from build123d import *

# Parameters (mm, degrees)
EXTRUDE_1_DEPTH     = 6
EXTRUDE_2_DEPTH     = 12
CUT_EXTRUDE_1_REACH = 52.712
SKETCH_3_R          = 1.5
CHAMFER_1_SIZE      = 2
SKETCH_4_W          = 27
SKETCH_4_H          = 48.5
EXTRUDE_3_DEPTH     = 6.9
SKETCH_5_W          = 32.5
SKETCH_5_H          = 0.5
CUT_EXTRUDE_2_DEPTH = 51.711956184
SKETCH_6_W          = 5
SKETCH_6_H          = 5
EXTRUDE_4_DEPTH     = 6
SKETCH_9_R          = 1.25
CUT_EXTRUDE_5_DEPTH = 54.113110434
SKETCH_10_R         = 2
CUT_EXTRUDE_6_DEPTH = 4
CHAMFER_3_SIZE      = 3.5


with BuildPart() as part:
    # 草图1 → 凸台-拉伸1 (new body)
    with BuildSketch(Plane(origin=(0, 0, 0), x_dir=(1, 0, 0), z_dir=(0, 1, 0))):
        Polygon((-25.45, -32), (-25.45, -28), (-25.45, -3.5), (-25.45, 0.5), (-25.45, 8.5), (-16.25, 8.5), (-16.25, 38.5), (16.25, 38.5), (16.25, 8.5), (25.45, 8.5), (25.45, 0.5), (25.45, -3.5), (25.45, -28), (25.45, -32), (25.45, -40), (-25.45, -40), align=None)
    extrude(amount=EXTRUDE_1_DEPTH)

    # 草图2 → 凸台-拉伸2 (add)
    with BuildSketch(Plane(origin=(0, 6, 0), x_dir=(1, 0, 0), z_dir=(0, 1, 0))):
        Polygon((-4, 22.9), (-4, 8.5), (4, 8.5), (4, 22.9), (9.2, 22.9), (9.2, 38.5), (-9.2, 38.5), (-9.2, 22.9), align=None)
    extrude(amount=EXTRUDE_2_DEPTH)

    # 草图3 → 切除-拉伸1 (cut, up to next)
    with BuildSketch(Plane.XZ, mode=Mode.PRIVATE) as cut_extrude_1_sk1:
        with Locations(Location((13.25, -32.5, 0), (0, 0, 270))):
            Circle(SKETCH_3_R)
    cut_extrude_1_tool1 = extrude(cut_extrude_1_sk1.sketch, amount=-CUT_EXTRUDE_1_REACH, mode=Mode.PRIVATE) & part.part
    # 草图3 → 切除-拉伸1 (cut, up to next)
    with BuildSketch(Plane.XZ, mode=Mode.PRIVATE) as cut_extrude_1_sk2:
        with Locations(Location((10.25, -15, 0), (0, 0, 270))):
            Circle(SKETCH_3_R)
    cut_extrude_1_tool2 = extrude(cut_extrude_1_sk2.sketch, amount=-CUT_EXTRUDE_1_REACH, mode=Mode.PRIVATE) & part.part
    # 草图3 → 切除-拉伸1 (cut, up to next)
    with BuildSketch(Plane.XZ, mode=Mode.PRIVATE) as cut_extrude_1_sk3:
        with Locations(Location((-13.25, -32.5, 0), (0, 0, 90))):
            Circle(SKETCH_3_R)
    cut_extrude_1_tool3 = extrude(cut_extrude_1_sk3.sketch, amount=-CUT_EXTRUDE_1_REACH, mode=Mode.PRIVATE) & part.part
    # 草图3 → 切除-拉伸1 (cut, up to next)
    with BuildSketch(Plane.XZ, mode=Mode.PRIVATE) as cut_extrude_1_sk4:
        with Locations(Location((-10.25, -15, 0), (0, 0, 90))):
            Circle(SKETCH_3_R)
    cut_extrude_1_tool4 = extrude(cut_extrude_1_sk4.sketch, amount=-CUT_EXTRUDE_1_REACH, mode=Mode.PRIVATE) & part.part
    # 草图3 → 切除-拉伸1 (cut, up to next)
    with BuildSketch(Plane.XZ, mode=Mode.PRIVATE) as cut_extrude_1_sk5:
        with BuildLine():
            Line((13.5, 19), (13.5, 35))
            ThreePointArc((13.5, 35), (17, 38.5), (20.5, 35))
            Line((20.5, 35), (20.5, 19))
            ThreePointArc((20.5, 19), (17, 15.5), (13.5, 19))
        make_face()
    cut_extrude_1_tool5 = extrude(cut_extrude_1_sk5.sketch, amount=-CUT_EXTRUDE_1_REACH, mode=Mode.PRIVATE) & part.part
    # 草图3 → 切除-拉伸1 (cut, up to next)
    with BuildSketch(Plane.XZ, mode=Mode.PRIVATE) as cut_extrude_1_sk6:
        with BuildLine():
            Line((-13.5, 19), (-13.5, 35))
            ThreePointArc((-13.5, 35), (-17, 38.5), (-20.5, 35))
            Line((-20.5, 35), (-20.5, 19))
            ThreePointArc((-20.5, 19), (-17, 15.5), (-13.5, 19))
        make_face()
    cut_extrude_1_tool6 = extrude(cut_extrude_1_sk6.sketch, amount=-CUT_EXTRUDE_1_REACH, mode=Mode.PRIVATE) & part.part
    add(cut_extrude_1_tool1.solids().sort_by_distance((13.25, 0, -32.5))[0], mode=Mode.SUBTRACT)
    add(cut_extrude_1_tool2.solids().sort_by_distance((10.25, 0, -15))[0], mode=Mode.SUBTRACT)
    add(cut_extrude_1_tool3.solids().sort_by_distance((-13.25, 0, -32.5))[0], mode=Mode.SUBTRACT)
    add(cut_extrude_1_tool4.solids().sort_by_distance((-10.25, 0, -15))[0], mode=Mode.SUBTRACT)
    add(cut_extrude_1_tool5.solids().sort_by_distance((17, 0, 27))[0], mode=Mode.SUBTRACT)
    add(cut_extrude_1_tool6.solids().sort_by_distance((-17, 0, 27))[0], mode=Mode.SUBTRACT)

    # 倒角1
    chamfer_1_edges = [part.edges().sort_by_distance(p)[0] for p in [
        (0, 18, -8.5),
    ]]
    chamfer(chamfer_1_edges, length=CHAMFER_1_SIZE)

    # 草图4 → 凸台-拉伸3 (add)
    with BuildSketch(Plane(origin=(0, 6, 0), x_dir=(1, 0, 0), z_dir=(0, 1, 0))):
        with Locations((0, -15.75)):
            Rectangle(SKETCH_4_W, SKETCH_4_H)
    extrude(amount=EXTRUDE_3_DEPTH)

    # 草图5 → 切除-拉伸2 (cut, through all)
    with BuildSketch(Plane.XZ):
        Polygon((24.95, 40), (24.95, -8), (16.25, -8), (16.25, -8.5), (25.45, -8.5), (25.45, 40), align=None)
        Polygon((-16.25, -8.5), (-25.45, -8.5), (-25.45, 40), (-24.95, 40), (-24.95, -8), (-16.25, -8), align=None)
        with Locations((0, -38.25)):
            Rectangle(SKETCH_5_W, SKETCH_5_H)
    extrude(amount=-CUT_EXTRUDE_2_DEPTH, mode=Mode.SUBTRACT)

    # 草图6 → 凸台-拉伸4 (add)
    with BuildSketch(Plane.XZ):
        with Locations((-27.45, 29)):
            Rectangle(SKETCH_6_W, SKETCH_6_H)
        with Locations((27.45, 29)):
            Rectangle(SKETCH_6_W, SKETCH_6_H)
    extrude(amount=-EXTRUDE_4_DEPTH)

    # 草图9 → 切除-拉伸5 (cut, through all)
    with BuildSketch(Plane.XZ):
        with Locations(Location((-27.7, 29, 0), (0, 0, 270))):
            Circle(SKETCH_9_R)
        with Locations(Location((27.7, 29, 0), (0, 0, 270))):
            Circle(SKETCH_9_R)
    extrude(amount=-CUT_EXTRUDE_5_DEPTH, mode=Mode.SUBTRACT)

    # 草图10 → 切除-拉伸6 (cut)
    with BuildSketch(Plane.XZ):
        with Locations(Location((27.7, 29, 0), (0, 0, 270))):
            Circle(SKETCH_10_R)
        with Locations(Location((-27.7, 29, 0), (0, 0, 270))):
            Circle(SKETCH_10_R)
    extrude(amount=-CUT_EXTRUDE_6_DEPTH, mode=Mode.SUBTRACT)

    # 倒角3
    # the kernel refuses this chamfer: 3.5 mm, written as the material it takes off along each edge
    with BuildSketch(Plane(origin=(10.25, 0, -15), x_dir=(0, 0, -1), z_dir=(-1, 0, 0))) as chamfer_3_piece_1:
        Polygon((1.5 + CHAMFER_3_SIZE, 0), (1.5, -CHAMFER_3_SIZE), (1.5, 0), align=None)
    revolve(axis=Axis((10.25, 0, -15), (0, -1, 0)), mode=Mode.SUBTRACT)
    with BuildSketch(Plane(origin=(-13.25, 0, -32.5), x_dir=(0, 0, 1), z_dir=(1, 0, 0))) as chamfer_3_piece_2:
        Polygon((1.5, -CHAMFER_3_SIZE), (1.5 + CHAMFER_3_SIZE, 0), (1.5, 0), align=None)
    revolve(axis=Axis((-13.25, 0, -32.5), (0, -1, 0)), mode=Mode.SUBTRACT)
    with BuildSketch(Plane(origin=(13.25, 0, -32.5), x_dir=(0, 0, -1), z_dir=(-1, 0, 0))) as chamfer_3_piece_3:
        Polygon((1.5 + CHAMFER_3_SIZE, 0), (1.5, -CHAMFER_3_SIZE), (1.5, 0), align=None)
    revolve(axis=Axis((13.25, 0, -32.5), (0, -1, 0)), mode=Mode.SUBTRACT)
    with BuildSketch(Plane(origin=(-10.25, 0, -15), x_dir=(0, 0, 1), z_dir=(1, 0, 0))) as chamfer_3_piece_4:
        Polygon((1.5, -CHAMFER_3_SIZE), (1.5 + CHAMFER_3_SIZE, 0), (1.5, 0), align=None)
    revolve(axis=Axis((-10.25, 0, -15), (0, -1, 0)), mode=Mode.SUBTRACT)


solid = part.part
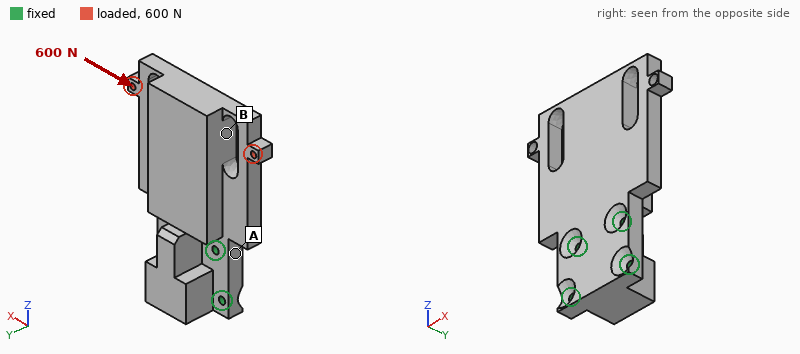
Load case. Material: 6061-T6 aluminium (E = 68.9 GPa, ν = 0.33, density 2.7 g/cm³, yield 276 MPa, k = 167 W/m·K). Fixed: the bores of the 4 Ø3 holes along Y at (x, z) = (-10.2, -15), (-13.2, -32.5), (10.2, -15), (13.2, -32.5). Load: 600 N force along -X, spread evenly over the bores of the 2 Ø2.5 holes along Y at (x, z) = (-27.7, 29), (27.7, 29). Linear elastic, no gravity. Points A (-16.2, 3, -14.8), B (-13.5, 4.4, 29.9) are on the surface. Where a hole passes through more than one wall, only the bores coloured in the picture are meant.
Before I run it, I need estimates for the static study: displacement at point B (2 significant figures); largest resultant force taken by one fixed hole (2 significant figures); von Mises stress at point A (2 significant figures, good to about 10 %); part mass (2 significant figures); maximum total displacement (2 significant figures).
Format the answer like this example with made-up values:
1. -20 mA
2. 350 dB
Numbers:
1. 22 µm
2. 970 N
3. 21 MPa
4. 86 g
5. 48 µm
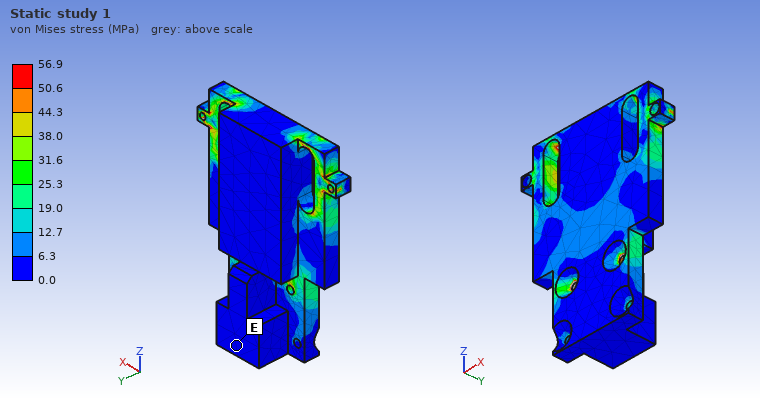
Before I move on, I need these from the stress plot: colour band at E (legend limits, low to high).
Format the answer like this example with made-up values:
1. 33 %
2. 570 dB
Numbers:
1. 0.0 to 6.3 MPa
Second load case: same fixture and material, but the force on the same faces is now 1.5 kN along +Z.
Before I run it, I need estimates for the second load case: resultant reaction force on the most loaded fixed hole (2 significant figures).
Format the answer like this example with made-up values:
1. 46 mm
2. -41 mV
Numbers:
1. 580 N
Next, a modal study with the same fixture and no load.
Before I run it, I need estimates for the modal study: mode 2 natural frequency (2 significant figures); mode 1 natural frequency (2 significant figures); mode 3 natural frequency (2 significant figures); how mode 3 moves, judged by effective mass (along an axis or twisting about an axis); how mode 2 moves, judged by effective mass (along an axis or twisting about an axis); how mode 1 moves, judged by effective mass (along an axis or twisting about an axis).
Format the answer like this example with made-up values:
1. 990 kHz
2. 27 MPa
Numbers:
1. 4500 Hz
2. 1800 Hz
3. 5200 Hz
4. twisting about Z
5. along X
6. along Y
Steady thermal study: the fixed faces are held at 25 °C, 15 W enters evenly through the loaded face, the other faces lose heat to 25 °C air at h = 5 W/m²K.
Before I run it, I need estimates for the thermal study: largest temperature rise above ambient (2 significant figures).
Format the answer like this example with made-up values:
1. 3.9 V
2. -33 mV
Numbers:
1. 41 K
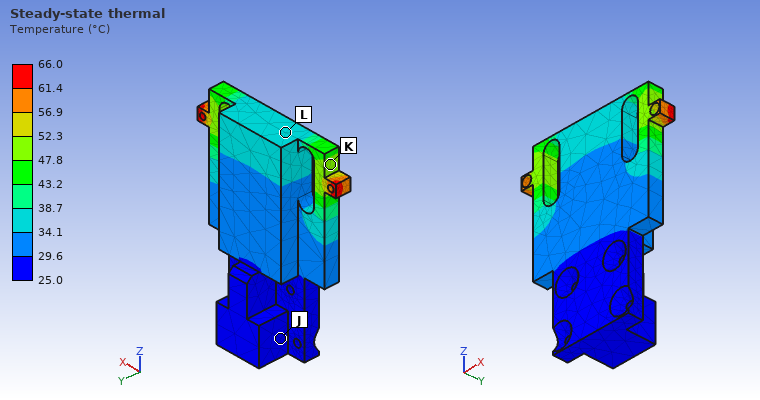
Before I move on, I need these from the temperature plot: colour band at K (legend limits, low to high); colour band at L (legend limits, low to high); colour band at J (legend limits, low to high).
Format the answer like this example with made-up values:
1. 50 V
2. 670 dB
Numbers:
1. 47.8 to 52.3 °C
2. 34.1 to 38.7 °C
3. 25.0 to 29.6 °C
